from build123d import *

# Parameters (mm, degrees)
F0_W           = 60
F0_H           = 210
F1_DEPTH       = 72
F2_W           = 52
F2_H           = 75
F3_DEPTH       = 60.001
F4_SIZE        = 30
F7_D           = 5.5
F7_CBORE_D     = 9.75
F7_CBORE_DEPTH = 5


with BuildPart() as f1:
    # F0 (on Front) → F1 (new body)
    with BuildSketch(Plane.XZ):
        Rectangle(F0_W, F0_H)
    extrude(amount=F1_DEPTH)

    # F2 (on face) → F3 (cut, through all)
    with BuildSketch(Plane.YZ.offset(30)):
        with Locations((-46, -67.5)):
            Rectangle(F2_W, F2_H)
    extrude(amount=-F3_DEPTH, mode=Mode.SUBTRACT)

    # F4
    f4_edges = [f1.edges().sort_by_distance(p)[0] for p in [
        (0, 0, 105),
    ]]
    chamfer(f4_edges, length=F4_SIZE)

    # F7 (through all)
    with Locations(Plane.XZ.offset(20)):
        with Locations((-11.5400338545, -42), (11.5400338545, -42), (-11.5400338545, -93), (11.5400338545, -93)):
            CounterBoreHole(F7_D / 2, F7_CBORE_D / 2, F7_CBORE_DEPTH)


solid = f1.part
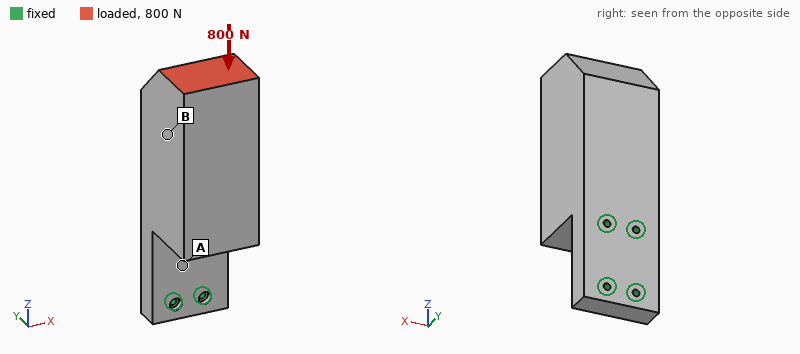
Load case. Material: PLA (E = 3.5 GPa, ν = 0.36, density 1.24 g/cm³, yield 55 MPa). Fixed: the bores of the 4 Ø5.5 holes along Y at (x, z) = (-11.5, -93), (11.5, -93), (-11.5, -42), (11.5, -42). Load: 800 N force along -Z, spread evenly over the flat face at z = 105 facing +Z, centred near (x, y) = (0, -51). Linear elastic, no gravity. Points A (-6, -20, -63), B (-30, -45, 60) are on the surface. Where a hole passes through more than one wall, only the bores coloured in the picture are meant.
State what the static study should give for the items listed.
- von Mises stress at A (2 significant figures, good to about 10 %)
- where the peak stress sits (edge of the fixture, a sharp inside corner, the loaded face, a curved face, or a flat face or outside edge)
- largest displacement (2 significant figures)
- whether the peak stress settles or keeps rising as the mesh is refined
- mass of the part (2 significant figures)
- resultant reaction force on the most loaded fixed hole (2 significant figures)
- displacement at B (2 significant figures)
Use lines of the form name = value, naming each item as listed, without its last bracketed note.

von Mises stress at A = 1.9 MPa
where the peak stress sits = edge of the fixture
largest displacement = 1.1 mm
whether the peak stress settles or keeps rising as the mesh is refined = keeps rising
mass of the part = 800 g
resultant reaction force on the most loaded fixed hole = 260 N
displacement at B = 0.72 mm
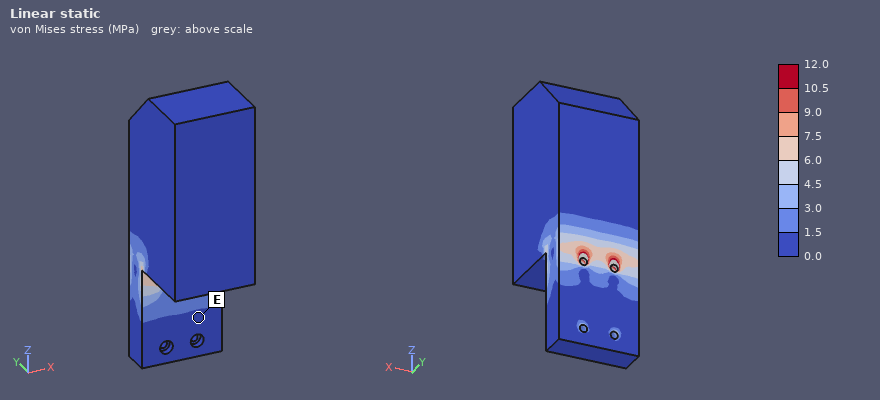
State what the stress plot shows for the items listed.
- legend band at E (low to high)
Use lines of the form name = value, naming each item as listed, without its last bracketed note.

legend band at E = 0.0 to 1.5 MPa
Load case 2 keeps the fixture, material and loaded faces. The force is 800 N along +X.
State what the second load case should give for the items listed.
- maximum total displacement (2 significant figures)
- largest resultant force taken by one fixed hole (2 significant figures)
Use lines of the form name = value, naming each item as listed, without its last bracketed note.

maximum total displacement = 0.87 mm
largest resultant force taken by one fixed hole = 2.8 kN
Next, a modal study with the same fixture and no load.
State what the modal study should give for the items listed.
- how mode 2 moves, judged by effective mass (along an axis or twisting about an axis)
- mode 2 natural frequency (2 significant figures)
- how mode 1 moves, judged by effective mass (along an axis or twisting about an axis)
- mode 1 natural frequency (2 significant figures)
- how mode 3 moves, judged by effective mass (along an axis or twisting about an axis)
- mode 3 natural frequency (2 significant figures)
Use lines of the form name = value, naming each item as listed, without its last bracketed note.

how mode 2 moves, judged by effective mass = along X
mode 2 natural frequency = 330 Hz
how mode 1 moves, judged by effective mass = along Y
mode 1 natural frequency = 150 Hz
how mode 3 moves, judged by effective mass = twisting about Z
mode 3 natural frequency = 670 Hz
